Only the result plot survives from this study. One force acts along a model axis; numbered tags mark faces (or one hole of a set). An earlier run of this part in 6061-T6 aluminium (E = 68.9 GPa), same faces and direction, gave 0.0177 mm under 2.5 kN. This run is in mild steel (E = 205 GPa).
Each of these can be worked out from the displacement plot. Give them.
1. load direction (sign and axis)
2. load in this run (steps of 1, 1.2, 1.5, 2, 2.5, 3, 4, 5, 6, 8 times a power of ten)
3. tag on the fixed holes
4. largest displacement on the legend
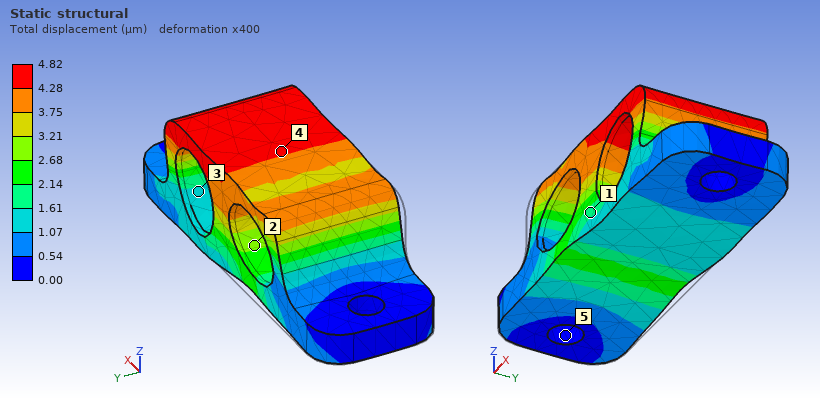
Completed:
+X
2 kN
5
4.82 µm
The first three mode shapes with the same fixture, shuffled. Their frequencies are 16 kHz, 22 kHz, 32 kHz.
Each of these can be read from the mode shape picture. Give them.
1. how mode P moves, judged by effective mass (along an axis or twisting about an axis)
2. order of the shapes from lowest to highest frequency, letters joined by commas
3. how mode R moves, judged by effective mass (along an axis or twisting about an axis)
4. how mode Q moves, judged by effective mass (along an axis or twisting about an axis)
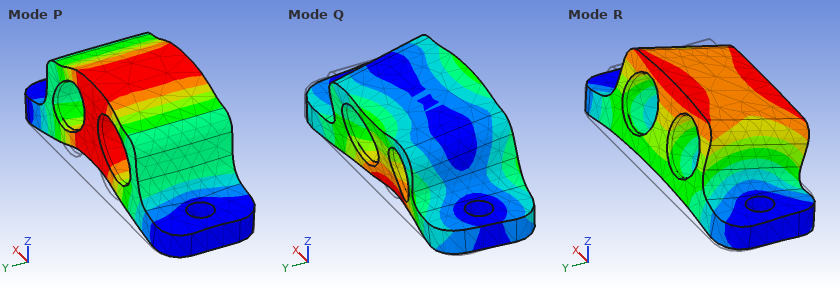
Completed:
along Z
R, P, Q
along Y
along Y
